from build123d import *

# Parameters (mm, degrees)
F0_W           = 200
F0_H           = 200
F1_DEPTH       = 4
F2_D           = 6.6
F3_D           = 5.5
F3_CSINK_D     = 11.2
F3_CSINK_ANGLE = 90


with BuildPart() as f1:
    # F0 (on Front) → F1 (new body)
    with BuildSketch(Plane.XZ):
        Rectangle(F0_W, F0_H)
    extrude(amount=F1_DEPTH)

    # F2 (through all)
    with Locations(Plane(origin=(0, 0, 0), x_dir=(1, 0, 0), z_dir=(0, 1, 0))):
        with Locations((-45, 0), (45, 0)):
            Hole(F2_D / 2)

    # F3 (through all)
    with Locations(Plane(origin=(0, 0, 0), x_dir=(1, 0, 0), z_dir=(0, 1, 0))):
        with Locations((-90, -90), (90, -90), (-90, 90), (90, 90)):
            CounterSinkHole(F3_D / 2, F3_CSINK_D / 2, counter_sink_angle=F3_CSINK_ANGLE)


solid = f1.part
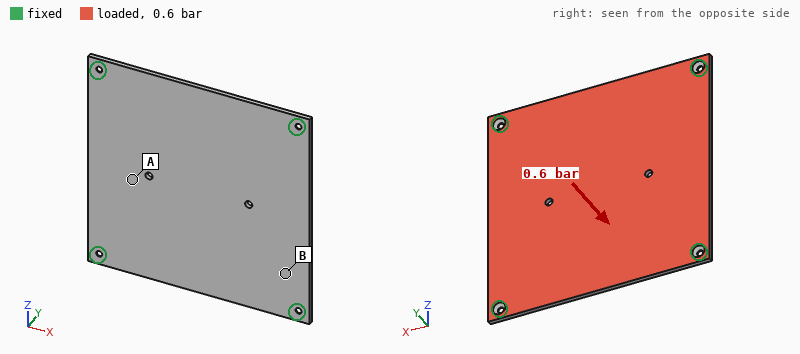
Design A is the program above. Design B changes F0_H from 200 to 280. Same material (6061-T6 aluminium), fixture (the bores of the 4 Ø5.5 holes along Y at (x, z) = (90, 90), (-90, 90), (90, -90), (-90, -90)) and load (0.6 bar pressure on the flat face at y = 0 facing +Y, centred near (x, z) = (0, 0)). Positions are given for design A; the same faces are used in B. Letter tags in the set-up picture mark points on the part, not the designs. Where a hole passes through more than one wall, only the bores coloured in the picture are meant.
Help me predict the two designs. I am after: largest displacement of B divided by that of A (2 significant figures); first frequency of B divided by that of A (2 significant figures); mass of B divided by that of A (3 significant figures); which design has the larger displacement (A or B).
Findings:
0.91
1.0
1.40
A
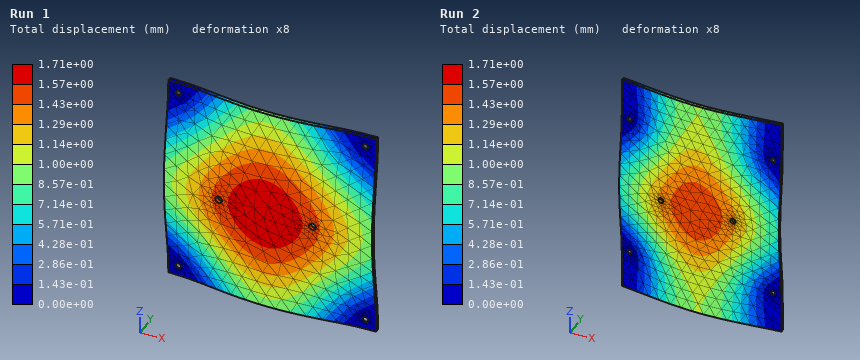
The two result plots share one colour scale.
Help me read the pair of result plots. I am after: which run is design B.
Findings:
Run 2
